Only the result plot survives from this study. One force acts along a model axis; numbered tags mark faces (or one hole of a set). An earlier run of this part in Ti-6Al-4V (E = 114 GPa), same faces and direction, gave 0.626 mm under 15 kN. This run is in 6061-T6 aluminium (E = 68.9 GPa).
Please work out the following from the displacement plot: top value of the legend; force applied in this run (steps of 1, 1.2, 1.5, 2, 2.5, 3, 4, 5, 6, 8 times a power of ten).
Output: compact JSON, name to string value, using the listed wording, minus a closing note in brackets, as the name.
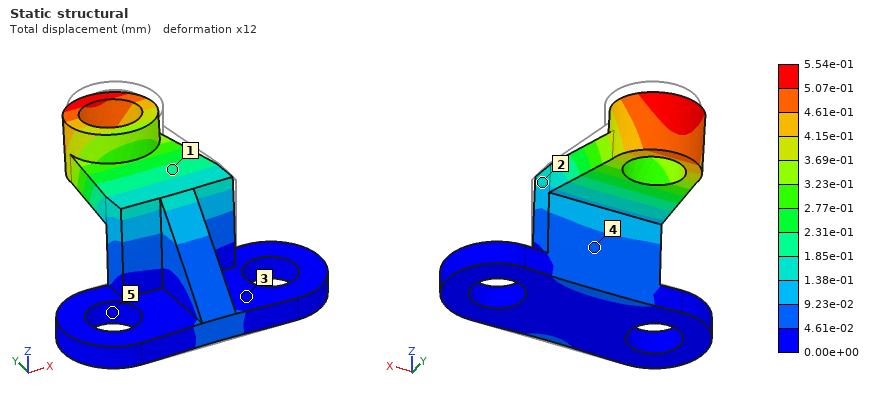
{"top value of the legend": "5.54e-01 mm", "force applied in this run": "8 kN"}
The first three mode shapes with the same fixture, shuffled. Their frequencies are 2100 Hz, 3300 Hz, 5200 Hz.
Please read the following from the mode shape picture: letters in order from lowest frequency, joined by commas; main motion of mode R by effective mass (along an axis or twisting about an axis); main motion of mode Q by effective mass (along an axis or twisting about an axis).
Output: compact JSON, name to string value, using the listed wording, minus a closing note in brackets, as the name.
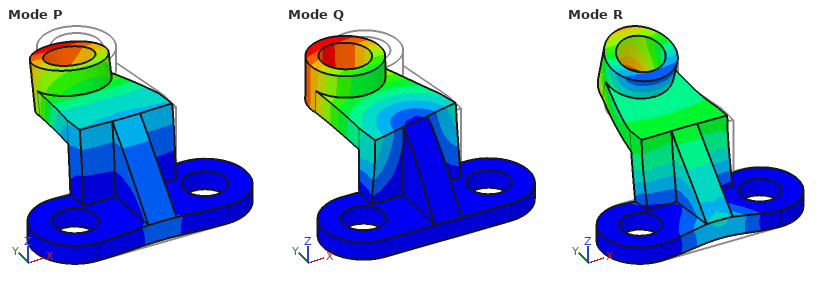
{"letters in order from lowest frequency, joined by commas": "P, Q, R", "main motion of mode R by effective mass": "along Y", "main motion of mode Q by effective mass": "along X"}
